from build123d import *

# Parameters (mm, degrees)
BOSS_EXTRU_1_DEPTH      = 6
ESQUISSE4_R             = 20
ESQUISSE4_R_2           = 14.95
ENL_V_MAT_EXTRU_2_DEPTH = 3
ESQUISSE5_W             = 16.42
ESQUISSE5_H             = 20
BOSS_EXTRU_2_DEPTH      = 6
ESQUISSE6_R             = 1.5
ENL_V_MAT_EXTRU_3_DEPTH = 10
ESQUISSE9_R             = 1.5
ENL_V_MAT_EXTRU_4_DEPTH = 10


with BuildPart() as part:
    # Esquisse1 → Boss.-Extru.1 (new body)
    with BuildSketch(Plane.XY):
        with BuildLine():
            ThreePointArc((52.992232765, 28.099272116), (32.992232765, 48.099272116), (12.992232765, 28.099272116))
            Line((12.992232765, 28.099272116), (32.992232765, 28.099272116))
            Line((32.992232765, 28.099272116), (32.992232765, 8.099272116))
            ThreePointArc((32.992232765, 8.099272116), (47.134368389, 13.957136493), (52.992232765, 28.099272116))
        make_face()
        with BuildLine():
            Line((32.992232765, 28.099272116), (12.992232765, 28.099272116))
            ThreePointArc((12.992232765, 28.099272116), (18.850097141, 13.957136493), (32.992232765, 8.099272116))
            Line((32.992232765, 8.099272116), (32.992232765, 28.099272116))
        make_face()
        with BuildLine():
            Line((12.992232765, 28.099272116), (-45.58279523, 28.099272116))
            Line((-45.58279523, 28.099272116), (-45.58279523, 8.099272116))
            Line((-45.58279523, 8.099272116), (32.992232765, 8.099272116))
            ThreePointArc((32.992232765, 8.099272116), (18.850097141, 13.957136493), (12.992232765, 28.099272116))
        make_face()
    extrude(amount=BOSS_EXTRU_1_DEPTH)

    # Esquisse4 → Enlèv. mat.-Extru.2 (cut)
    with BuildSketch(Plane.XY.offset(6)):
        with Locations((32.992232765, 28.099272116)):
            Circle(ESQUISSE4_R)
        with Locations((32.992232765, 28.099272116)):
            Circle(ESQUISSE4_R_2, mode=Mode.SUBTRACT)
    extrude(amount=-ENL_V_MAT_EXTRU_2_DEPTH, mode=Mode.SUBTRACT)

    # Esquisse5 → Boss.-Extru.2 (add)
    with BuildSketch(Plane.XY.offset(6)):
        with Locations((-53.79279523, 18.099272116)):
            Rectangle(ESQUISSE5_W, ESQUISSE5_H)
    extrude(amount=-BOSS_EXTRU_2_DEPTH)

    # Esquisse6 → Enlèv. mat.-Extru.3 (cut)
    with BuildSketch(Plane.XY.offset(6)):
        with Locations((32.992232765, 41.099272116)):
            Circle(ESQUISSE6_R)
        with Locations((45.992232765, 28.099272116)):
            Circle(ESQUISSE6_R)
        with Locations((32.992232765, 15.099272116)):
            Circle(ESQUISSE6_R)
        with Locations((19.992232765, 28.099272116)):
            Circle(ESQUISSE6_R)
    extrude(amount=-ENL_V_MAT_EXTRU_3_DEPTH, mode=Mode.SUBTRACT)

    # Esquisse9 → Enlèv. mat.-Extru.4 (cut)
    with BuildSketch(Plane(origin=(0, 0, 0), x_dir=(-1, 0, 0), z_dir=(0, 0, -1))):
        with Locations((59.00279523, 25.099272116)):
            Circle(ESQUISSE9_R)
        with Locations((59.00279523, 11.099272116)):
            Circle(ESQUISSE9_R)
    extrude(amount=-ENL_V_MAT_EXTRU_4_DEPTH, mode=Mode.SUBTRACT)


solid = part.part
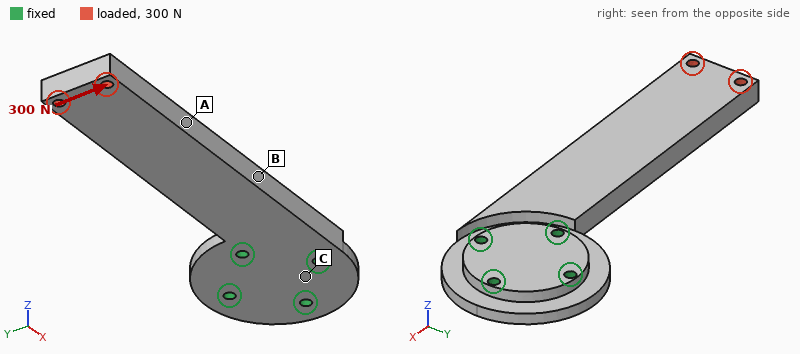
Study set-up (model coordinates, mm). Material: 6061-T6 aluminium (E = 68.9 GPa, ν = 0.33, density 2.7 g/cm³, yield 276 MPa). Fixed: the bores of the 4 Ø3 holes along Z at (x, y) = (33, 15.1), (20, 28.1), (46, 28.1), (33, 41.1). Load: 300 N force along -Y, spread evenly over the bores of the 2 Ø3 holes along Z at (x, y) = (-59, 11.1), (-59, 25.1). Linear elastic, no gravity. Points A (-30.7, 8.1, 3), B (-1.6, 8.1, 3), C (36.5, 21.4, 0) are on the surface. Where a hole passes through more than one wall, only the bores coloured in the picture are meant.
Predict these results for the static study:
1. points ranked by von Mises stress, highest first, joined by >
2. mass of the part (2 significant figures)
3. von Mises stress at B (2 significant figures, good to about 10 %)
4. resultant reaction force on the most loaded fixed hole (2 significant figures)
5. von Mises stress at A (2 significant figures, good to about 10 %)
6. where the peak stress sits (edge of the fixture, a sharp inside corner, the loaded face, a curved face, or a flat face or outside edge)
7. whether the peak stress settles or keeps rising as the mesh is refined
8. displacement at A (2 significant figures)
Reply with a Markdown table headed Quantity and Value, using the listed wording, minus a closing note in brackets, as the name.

| Quantity | Value |
|---|---|
| points ranked by von Mises stress, highest first, joined by > | B > A > C |
| mass of the part | 41 g |
| von Mises stress at B | 44 MPa |
| resultant reaction force on the most loaded fixed hole | 1.2 kN |
| von Mises stress at A | 21 MPa |
| where the peak stress sits | a sharp inside corner |
| whether the peak stress settles or keeps rising as the mesh is refined | keeps rising |
| displacement at A | 0.16 mm |
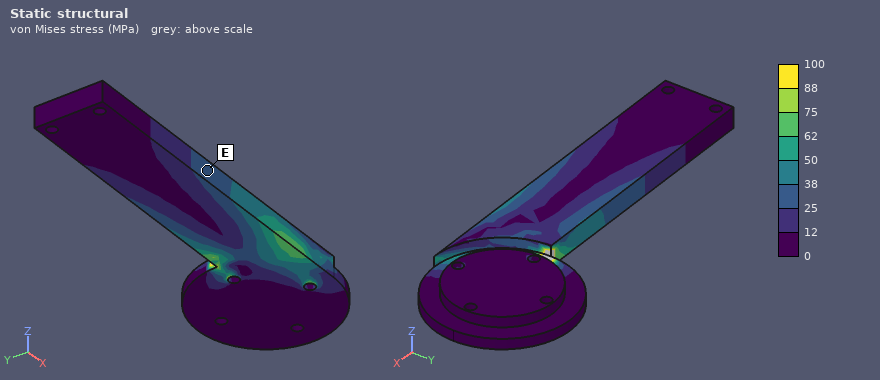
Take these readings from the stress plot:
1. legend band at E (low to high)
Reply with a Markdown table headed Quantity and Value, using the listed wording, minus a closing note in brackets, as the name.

| Quantity | Value |
|---|---|
| legend band at E | 25 to 38 MPa |
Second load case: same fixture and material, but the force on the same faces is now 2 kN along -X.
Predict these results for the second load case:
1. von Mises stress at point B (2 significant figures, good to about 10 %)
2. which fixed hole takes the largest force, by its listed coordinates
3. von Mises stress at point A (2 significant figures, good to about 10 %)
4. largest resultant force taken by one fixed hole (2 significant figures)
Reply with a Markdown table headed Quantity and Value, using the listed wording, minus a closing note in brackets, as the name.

| Quantity | Value |
|---|---|
| von Mises stress at point B | 17 MPa |
| which fixed hole takes the largest force, by its listed coordinates | (33, 15.1) |
| von Mises stress at point A | 17 MPa |
| largest resultant force taken by one fixed hole | 1.1 kN |
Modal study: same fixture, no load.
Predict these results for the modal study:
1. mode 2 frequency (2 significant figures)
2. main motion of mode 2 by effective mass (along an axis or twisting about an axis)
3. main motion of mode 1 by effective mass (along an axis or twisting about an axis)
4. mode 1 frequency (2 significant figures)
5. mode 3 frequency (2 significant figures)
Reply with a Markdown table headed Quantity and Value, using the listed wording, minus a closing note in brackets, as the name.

| Quantity | Value |
|---|---|
| mode 2 frequency | 2000 Hz |
| main motion of mode 2 by effective mass | along Y |
| main motion of mode 1 by effective mass | along Z |
| mode 1 frequency | 460 Hz |
| mode 3 frequency | 3300 Hz |
